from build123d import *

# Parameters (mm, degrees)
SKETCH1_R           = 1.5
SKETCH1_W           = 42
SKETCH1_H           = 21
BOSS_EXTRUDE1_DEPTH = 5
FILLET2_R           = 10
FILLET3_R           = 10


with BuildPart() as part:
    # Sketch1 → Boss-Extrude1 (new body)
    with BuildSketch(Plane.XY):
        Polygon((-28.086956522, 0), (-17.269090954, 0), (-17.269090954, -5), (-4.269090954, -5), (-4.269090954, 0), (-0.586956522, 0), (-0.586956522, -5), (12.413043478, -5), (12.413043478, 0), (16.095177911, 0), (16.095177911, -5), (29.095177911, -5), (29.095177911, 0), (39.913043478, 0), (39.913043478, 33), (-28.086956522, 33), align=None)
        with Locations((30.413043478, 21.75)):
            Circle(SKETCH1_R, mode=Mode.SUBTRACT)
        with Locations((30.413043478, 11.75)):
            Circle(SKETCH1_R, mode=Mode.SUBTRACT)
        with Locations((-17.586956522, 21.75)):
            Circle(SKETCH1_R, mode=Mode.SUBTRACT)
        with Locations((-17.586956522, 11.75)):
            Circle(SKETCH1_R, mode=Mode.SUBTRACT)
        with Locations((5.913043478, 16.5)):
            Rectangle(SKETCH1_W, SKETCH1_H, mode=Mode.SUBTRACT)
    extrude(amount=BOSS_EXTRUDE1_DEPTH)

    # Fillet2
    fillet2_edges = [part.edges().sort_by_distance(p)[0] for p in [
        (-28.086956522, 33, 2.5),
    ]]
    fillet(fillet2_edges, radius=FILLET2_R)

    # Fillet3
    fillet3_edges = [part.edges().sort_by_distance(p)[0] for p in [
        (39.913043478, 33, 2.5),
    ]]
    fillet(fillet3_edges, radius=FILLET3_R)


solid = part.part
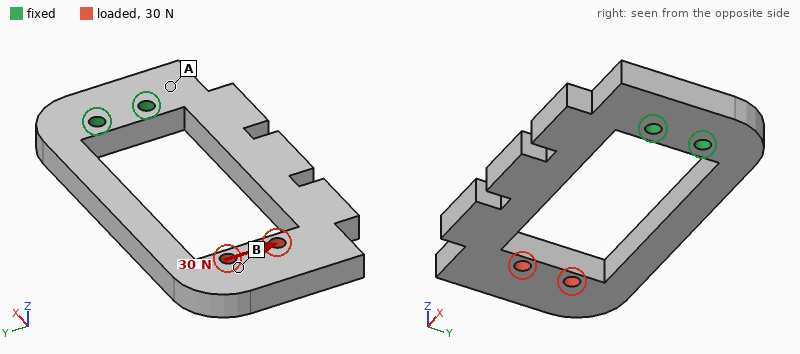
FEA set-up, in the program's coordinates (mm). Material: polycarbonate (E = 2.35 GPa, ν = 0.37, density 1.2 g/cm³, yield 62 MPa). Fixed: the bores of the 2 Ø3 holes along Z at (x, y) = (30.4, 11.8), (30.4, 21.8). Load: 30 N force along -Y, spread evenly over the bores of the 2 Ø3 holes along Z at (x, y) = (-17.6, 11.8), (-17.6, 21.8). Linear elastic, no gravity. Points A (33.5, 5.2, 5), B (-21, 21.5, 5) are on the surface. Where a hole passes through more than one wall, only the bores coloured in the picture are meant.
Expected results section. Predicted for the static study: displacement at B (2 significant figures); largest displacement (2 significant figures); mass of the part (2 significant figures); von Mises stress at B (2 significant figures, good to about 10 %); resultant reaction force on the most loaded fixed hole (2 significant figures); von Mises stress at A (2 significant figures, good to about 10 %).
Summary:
0.75 mm
0.79 mm
8.9 g
1.7 MPa
100 N
3.6 MPa
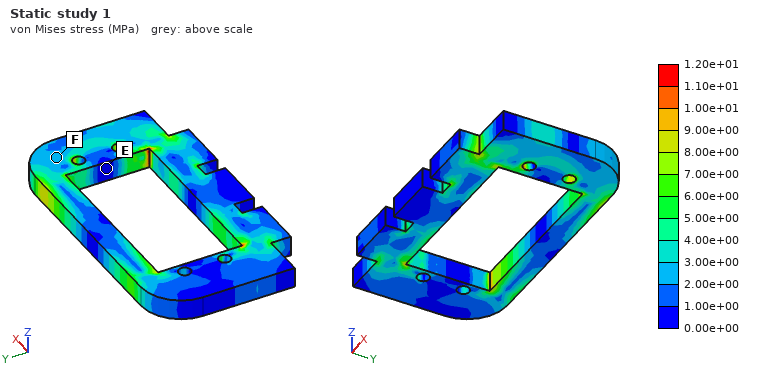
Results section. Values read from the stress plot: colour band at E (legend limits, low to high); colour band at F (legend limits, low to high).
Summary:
0.00e+00 to 1.00e+00 MPa
2.00e+00 to 3.00e+00 MPa
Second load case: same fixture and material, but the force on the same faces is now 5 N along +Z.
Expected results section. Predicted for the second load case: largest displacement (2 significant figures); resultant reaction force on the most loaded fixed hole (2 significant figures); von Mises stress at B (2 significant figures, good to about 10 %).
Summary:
0.92 mm
2.6 N
0.48 MPa
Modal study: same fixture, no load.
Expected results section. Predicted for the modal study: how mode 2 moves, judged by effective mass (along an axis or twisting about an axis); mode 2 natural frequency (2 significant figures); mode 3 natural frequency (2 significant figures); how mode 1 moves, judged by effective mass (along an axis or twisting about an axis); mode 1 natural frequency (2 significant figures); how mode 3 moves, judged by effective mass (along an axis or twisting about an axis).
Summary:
along Y
510 Hz
640 Hz
along Z
210 Hz
twisting about X
